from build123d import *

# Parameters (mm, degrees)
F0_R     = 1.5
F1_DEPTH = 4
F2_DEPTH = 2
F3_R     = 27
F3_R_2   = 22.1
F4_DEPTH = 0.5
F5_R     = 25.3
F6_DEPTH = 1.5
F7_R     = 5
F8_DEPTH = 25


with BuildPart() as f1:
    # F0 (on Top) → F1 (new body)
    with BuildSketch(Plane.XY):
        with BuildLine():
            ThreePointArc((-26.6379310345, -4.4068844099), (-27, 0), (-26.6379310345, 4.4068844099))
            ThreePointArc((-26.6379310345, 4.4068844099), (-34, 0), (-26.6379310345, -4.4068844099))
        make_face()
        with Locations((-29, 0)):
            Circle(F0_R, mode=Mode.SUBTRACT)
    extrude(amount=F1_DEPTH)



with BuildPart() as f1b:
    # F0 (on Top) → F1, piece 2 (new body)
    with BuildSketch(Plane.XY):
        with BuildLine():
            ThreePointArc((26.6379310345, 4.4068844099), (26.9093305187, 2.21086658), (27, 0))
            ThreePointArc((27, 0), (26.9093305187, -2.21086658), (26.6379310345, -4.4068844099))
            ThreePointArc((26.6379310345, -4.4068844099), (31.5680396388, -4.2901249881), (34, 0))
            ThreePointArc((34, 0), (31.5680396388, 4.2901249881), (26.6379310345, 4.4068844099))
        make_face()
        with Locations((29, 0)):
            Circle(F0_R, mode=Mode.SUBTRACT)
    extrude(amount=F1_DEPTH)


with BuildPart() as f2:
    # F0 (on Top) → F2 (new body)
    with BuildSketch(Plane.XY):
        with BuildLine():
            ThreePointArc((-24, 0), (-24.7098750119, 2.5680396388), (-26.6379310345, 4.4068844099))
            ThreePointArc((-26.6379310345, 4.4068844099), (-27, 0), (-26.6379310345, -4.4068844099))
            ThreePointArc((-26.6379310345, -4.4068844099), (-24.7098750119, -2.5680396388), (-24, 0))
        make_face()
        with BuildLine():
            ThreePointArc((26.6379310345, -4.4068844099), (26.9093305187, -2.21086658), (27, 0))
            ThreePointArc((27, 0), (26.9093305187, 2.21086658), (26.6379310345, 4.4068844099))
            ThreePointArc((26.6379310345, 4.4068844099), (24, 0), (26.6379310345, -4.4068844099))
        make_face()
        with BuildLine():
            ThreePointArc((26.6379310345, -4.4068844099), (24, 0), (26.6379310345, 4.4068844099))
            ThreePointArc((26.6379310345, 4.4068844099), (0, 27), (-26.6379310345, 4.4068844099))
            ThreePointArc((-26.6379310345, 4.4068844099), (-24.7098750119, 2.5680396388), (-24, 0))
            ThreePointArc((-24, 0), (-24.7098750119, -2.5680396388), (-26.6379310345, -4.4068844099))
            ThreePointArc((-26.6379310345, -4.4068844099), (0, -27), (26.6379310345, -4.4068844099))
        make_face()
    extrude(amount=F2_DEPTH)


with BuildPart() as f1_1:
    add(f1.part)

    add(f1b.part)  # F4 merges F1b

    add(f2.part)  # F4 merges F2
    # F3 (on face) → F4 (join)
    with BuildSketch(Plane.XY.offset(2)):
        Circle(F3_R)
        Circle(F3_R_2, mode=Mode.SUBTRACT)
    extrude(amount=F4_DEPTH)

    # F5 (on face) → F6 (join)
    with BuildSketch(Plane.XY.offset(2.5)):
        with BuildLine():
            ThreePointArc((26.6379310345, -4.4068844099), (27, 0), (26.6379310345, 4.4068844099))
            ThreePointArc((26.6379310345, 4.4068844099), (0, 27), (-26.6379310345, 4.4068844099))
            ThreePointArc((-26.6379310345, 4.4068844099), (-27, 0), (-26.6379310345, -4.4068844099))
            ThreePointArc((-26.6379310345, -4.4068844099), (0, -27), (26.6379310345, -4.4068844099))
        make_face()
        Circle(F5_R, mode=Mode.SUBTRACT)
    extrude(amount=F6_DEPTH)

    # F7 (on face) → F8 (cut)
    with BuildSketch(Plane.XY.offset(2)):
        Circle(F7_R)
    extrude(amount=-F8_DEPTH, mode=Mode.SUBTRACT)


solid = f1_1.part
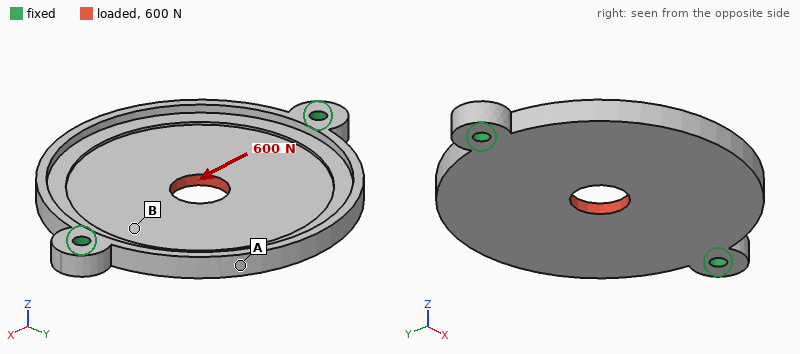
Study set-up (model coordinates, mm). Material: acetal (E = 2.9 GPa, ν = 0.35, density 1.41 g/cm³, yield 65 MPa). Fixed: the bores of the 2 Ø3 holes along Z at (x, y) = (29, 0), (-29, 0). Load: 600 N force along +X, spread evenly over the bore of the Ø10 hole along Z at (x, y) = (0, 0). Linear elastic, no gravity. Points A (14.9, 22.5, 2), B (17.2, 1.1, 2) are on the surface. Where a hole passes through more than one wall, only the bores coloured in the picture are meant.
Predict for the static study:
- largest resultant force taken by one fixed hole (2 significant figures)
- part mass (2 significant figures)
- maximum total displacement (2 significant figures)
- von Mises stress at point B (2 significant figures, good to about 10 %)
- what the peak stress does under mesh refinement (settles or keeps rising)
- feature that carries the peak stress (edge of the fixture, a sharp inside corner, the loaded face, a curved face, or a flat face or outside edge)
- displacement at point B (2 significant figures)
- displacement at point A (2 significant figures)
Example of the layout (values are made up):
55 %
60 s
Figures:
300 N
8.0 g
95 µm
12 MPa
keeps rising
edge of the fixture
57 µm
70 µm
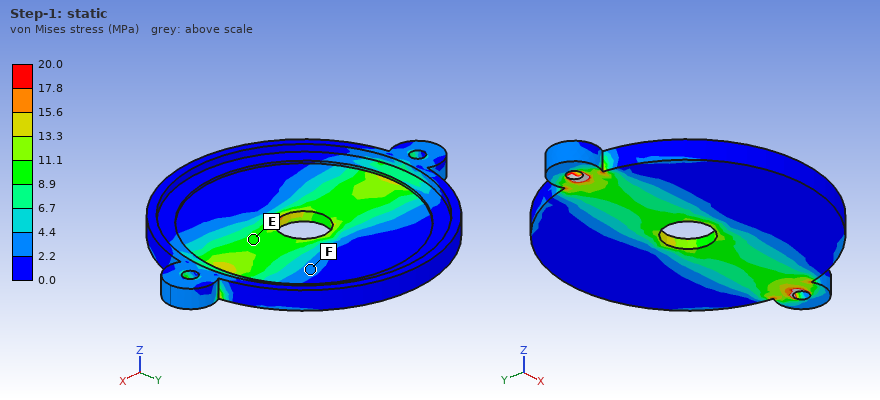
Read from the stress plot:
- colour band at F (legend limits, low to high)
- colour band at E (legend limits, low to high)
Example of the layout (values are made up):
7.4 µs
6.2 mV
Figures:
2.2 to 4.4 MPa
8.9 to 11.1 MPa
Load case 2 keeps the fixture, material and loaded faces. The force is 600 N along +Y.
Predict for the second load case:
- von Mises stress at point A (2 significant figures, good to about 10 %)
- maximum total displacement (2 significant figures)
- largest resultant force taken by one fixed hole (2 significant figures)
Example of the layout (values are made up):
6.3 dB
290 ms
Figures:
5.2 MPa
0.53 mm
300 N
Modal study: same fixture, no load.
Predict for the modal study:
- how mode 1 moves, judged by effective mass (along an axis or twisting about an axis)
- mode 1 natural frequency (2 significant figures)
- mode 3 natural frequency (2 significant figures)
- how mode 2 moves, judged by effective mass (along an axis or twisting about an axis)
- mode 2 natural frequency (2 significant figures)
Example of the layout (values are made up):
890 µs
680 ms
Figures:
twisting about X
620 Hz
1800 Hz
along Z
740 Hz
